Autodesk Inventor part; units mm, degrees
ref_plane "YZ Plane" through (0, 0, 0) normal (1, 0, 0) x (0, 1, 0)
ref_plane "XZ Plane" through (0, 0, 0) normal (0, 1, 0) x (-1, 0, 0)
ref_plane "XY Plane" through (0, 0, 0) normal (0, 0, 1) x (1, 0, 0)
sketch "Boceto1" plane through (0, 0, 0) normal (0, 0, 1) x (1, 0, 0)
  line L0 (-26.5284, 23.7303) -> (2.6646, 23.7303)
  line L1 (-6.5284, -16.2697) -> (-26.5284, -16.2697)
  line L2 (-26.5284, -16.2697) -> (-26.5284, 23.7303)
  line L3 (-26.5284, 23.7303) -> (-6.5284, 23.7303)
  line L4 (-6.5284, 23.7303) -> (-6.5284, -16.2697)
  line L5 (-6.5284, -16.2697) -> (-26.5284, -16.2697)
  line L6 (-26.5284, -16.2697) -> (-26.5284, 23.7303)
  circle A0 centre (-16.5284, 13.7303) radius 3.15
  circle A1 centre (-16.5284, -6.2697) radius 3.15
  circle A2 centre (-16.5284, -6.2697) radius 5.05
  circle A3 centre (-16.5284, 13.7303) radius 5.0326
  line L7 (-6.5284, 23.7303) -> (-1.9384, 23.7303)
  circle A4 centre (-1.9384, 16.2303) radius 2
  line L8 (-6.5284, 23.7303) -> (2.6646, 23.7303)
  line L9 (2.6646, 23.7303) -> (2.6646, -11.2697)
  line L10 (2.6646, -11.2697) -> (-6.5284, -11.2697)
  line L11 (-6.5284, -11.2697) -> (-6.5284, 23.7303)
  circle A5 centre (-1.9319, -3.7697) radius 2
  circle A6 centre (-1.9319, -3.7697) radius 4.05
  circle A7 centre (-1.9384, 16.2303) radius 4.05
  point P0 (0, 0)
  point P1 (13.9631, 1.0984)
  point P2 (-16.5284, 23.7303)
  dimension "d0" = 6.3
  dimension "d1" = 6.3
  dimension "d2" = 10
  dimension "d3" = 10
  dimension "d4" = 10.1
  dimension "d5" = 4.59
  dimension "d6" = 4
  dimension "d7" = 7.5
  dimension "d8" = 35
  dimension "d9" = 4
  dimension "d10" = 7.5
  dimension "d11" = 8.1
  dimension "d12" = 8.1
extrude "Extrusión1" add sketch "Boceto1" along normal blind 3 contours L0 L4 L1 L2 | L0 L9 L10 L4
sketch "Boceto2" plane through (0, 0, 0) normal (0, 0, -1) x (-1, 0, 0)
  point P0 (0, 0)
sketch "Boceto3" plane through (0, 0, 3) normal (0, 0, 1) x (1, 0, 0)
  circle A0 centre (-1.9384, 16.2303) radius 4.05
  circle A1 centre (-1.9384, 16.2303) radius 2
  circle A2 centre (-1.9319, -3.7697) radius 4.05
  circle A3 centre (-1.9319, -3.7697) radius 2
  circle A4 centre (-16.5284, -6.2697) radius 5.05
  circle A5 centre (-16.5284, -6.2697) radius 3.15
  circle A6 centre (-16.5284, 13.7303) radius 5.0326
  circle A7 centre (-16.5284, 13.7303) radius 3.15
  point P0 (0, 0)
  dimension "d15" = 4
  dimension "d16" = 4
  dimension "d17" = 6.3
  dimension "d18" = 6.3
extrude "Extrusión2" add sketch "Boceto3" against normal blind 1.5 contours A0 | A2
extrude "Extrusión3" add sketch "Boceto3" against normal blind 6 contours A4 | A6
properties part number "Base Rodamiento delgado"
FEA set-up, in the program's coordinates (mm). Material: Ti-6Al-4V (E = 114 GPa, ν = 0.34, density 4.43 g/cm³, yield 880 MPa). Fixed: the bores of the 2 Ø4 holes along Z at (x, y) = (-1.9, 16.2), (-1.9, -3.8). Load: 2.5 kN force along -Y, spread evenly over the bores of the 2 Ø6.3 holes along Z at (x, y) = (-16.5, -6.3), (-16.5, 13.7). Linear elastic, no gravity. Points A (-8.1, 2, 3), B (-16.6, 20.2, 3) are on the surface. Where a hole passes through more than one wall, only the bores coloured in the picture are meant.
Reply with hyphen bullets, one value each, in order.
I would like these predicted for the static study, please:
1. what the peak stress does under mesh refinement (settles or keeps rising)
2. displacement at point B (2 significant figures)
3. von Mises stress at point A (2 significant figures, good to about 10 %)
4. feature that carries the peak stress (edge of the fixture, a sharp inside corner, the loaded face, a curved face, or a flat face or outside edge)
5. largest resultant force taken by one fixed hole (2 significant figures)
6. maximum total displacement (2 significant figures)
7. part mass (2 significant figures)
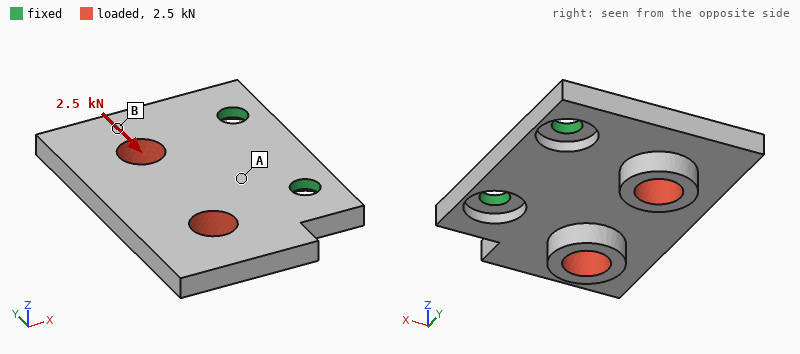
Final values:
- keeps rising
- 26 µm
- 59 MPa
- edge of the fixture
- 2.0 kN
- 61 µm
- 15 g
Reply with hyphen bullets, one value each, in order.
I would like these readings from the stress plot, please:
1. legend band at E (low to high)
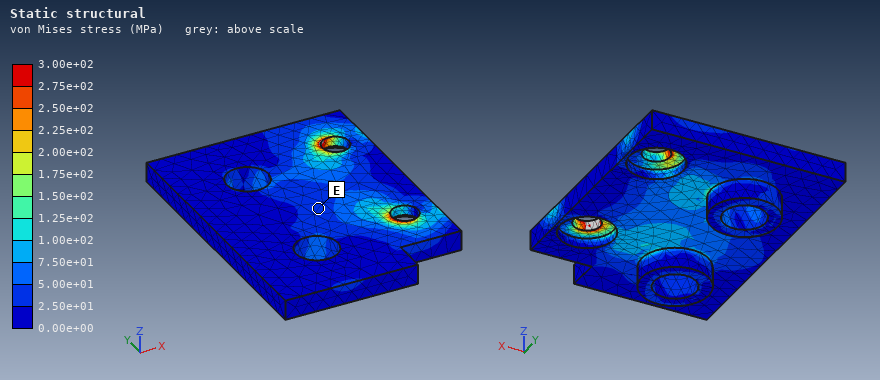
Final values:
- 2.50e+01 to 5.00e+01 MPa
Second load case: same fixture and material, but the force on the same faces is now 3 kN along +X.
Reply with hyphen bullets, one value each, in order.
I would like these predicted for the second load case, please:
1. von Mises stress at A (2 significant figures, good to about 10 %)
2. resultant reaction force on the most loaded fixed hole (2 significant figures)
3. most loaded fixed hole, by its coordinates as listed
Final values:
- 79 MPa
- 1.8 kN
- (-1.9, -3.8)
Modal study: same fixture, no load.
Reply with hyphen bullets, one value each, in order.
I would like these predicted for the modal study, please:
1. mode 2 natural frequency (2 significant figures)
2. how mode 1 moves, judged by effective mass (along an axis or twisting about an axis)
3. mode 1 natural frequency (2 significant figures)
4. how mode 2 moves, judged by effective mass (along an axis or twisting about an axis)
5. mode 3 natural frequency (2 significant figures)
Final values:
- 5300 Hz
- along Z
- 2700 Hz
- twisting about X
- 12 kHz
